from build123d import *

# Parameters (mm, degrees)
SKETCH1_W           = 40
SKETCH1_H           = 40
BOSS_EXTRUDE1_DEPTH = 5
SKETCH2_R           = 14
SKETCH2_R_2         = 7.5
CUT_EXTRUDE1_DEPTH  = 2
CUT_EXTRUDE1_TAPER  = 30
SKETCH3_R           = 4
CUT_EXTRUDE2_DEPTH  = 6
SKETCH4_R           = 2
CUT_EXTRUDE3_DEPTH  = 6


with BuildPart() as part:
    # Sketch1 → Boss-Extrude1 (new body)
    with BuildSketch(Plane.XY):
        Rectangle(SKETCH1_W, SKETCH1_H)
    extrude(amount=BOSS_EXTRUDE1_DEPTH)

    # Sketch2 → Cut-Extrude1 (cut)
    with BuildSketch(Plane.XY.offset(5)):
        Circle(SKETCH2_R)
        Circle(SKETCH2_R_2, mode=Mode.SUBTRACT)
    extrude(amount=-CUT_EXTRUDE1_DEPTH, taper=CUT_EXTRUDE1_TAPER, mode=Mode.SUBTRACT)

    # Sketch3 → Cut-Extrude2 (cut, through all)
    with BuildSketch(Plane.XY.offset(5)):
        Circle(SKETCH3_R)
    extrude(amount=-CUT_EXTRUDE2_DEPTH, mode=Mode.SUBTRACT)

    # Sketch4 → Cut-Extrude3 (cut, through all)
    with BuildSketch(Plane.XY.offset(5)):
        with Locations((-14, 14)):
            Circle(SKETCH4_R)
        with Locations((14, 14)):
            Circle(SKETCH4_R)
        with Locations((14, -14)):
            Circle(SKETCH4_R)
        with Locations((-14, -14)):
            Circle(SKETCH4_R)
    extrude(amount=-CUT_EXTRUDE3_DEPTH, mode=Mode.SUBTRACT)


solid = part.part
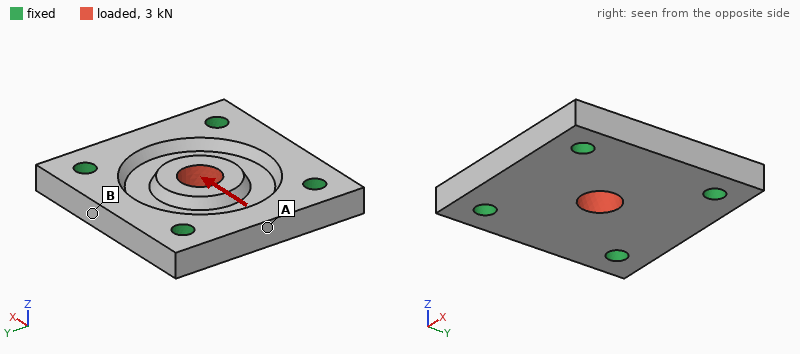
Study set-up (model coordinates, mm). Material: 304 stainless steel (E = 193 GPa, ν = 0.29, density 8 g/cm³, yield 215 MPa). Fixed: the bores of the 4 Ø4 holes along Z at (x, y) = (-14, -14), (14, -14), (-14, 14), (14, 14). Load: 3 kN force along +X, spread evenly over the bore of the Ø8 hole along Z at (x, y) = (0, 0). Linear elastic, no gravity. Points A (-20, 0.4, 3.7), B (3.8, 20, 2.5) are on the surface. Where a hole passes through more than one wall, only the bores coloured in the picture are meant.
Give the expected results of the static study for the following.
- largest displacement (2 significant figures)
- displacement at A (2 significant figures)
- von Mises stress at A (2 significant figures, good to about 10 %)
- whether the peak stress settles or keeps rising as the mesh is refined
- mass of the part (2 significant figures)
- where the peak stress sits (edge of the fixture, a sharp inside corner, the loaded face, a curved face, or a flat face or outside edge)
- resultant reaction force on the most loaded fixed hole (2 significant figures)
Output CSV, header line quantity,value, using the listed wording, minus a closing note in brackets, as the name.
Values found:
quantity,value
largest displacement,3.1 µm
displacement at A,1.1 µm
von Mises stress at A,13 MPa
whether the peak stress settles or keeps rising as the mesh is refined,keeps rising
mass of the part,54 g
where the peak stress sits,edge of the fixture
resultant reaction force on the most loaded fixed hole,800 N
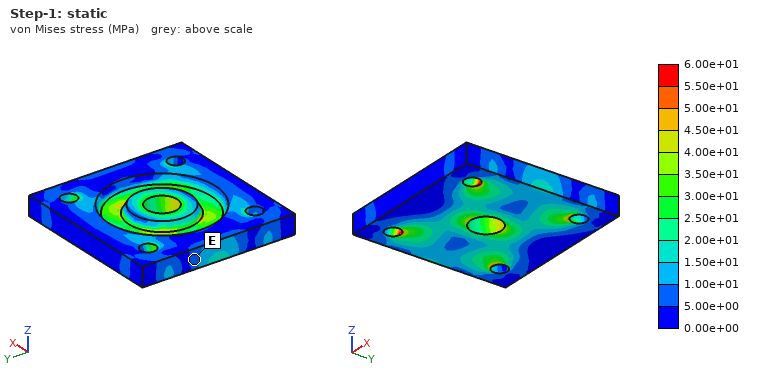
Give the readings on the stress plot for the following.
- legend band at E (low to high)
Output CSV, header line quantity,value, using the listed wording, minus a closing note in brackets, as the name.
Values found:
quantity,value
legend band at E,5.00e+00 to 1.00e+01 MPa
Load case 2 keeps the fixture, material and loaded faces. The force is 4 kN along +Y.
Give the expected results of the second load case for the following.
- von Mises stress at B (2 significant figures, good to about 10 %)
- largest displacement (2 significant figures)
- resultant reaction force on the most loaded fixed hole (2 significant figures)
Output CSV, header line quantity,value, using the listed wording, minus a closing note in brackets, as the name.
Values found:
quantity,value
von Mises stress at B,16 MPa
largest displacement,4.1 µm
resultant reaction force on the most loaded fixed hole,1.1 kN
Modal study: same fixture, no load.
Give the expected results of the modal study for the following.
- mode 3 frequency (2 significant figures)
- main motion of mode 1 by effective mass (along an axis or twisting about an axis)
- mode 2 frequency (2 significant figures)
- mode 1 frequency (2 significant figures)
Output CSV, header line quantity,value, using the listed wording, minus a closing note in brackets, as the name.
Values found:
quantity,value
mode 3 frequency,30 kHz
main motion of mode 1 by effective mass,along Z
mode 2 frequency,30 kHz
mode 1 frequency,22 kHz
